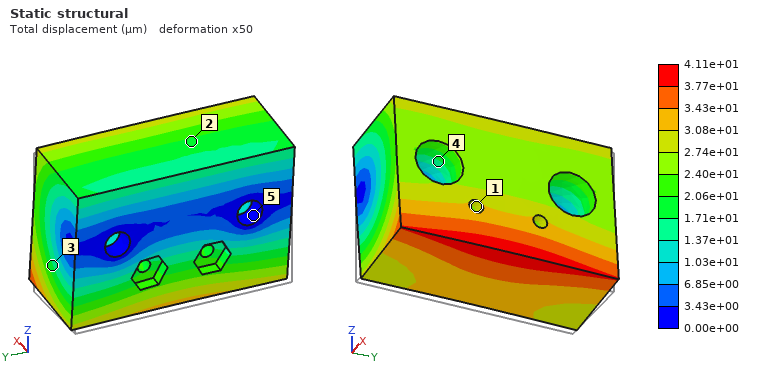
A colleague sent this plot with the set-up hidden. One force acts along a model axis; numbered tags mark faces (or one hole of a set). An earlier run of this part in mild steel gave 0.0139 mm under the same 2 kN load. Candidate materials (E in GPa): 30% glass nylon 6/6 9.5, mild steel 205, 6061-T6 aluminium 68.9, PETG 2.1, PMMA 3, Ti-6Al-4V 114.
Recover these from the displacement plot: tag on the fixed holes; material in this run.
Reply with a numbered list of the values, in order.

1. 5
2. 6061-T6 aluminium
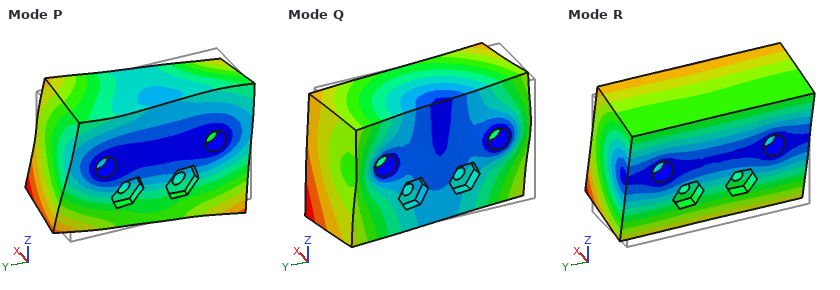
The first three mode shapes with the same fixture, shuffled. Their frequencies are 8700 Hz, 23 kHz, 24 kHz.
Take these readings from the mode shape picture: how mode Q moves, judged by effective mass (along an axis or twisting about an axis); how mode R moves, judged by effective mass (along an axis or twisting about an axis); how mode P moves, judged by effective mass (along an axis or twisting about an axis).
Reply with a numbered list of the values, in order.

1. along Y
2. along Z
3. twisting about X
